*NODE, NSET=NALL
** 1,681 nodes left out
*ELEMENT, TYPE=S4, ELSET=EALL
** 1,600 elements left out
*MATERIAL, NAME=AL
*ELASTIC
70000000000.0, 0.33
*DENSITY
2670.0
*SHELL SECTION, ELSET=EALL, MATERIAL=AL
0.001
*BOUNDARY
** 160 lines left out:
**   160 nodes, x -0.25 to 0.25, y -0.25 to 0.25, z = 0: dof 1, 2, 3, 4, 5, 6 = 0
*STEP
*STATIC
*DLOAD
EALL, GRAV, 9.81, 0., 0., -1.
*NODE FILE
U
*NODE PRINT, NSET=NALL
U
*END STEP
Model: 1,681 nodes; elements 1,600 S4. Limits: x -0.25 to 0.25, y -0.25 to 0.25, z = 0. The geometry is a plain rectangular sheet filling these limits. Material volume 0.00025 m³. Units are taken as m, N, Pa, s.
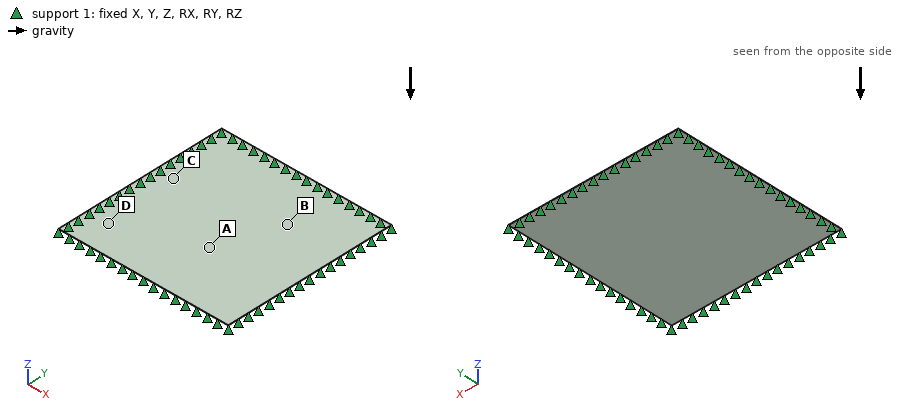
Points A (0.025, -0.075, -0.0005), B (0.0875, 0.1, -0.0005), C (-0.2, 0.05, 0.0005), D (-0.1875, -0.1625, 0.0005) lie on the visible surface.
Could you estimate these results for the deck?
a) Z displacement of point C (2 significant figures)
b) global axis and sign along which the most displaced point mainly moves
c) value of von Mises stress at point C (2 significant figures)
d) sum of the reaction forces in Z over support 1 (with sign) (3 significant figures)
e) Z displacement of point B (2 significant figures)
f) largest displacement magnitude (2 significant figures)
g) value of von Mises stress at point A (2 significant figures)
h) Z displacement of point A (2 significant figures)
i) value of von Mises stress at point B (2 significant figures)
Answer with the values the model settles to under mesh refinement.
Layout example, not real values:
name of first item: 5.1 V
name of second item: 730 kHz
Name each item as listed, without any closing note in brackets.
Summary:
Z displacement of point C: -4.3e-05 m
global axis and sign along which the most displaced point mainly moves: -Z
value of von Mises stress at point C: 5.8e+05 Pa
sum of the reaction forces in Z over support 1 (with sign): 6.55 N
Z displacement of point B: -1.8e-04 m
largest displacement magnitude: 3.1e-04 m
value of von Mises stress at point A: 7.6e+05 Pa
Z displacement of point A: -2.6e-04 m
value of von Mises stress at point B: 6.0e+05 Pa
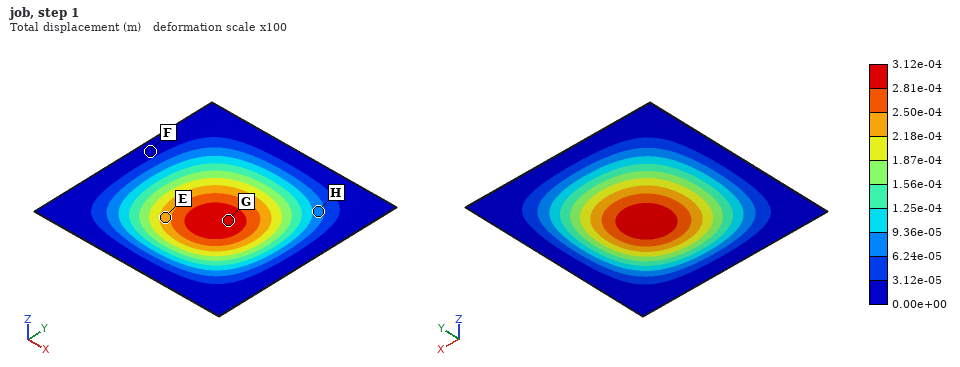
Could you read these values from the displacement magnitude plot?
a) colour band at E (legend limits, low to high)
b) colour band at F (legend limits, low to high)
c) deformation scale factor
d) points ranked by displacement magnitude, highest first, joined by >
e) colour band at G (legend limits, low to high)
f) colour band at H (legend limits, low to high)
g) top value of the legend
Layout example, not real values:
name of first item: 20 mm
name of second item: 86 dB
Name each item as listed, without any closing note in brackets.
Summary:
colour band at E: 2.18e-04 to 2.50e-04 m
colour band at F: 0.00e+00 to 3.12e-05 m
deformation scale factor: 100
points ranked by displacement magnitude, highest first, joined by >: G > E > H > F
colour band at G: 2.81e-04 to 3.12e-04 m
colour band at H: 6.24e-05 to 9.36e-05 m
top value of the legend: 3.12e-04 m
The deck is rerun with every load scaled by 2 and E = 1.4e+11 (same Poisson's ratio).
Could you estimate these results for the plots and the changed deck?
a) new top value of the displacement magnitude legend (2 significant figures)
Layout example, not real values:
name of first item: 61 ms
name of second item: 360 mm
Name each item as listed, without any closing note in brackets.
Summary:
new top value of the displacement magnitude legend: 3.1e-04 m
